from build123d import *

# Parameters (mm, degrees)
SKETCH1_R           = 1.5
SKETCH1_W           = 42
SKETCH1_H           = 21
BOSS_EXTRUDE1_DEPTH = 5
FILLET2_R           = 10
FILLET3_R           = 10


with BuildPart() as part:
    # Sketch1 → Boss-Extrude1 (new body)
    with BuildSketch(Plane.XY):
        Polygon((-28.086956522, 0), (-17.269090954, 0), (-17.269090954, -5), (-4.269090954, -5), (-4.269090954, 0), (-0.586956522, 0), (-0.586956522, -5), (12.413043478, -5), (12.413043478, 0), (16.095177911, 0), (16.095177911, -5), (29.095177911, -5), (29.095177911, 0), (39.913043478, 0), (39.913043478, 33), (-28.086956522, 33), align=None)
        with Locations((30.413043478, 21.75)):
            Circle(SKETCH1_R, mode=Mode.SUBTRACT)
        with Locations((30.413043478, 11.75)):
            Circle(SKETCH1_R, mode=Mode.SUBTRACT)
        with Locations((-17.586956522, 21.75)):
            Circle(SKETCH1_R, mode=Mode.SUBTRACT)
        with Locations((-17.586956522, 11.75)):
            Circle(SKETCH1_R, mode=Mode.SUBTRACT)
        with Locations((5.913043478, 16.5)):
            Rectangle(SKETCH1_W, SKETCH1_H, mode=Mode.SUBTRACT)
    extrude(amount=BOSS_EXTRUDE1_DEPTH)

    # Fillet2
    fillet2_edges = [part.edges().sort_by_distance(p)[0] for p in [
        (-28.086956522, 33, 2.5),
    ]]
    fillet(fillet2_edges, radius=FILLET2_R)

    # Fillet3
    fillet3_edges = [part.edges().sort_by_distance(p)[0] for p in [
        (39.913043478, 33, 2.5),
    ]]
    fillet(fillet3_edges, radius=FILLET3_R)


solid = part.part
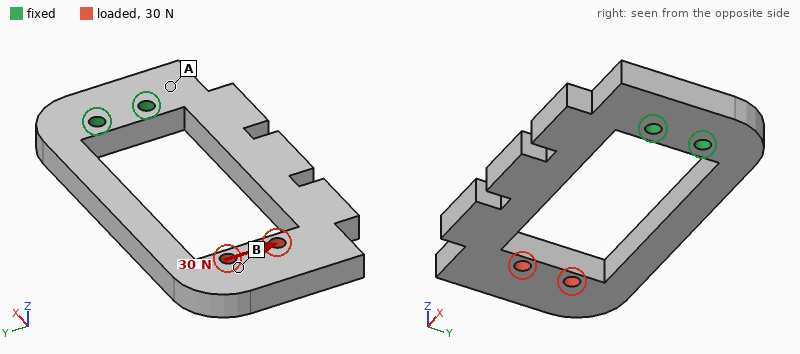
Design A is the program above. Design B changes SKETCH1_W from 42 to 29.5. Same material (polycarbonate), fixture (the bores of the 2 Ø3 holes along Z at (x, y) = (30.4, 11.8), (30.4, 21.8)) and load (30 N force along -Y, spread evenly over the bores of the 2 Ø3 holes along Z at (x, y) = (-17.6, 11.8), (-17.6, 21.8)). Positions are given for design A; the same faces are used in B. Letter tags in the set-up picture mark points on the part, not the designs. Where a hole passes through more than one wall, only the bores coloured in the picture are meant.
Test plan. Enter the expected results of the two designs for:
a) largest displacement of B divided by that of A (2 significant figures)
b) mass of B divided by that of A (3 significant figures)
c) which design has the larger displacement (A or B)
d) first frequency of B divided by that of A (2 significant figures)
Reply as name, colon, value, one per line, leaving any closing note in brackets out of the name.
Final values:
largest displacement of B divided by that of A: 0.47
mass of B divided by that of A: 1.18
which design has the larger displacement: A
first frequency of B divided by that of A: 1.1
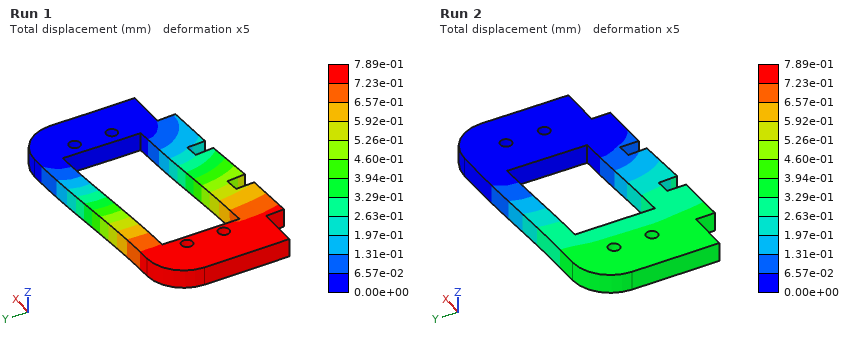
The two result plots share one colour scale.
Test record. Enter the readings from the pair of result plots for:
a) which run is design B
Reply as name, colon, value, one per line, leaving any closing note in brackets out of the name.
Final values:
which run is design B: Run 2
